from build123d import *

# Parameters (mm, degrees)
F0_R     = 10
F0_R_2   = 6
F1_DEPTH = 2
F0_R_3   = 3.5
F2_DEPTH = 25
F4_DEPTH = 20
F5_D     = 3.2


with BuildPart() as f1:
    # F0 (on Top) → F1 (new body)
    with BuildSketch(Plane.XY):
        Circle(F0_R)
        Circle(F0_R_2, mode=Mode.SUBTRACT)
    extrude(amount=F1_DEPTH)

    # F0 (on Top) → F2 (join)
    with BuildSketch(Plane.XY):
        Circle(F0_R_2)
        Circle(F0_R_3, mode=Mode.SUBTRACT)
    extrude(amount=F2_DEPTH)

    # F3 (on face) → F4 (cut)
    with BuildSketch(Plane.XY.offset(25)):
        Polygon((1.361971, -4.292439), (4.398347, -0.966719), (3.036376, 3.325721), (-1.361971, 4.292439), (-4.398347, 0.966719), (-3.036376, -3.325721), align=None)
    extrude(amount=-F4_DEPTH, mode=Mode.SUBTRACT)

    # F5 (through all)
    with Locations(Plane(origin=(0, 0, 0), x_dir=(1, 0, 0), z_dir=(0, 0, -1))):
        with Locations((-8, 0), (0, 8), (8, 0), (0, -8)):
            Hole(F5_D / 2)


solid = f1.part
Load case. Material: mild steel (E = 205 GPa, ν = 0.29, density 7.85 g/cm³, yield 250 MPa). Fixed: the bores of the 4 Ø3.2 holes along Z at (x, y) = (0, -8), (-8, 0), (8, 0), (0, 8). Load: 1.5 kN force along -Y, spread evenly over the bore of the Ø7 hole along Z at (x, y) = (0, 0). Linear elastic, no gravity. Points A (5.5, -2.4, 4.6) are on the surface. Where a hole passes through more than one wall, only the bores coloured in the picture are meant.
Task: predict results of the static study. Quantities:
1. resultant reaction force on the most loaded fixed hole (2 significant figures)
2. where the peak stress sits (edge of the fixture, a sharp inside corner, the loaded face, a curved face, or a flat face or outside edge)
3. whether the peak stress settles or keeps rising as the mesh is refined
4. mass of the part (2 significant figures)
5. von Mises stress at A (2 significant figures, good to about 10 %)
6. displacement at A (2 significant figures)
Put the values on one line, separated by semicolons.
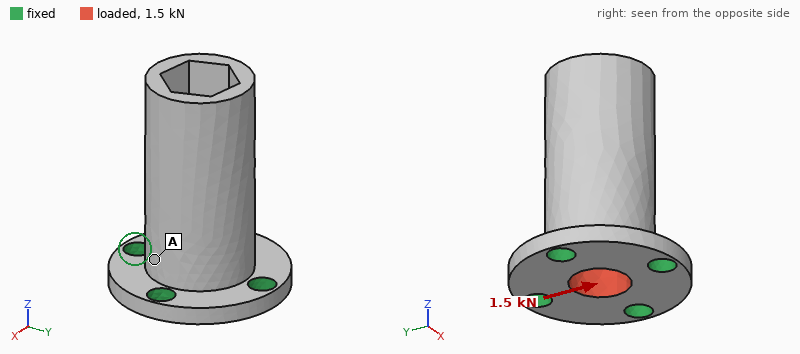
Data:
480 N; edge of the fixture; keeps rising; 15 g; 11 MPa; 0.90 µm
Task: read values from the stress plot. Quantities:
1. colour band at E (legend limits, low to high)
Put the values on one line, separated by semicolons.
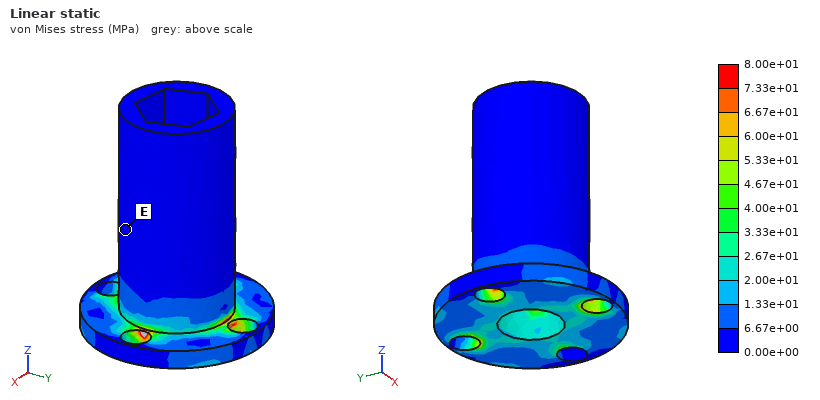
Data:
0.00e+00 to 6.67e+00 MPa
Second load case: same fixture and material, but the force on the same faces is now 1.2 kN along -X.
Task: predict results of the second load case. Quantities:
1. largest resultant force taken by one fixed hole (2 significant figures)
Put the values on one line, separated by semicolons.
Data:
380 N
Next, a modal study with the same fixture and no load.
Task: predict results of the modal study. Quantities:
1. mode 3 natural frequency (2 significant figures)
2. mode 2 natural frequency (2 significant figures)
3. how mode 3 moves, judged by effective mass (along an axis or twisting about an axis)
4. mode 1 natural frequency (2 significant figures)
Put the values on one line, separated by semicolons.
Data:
33 kHz; 12 kHz; twisting about Z; 12 kHz
